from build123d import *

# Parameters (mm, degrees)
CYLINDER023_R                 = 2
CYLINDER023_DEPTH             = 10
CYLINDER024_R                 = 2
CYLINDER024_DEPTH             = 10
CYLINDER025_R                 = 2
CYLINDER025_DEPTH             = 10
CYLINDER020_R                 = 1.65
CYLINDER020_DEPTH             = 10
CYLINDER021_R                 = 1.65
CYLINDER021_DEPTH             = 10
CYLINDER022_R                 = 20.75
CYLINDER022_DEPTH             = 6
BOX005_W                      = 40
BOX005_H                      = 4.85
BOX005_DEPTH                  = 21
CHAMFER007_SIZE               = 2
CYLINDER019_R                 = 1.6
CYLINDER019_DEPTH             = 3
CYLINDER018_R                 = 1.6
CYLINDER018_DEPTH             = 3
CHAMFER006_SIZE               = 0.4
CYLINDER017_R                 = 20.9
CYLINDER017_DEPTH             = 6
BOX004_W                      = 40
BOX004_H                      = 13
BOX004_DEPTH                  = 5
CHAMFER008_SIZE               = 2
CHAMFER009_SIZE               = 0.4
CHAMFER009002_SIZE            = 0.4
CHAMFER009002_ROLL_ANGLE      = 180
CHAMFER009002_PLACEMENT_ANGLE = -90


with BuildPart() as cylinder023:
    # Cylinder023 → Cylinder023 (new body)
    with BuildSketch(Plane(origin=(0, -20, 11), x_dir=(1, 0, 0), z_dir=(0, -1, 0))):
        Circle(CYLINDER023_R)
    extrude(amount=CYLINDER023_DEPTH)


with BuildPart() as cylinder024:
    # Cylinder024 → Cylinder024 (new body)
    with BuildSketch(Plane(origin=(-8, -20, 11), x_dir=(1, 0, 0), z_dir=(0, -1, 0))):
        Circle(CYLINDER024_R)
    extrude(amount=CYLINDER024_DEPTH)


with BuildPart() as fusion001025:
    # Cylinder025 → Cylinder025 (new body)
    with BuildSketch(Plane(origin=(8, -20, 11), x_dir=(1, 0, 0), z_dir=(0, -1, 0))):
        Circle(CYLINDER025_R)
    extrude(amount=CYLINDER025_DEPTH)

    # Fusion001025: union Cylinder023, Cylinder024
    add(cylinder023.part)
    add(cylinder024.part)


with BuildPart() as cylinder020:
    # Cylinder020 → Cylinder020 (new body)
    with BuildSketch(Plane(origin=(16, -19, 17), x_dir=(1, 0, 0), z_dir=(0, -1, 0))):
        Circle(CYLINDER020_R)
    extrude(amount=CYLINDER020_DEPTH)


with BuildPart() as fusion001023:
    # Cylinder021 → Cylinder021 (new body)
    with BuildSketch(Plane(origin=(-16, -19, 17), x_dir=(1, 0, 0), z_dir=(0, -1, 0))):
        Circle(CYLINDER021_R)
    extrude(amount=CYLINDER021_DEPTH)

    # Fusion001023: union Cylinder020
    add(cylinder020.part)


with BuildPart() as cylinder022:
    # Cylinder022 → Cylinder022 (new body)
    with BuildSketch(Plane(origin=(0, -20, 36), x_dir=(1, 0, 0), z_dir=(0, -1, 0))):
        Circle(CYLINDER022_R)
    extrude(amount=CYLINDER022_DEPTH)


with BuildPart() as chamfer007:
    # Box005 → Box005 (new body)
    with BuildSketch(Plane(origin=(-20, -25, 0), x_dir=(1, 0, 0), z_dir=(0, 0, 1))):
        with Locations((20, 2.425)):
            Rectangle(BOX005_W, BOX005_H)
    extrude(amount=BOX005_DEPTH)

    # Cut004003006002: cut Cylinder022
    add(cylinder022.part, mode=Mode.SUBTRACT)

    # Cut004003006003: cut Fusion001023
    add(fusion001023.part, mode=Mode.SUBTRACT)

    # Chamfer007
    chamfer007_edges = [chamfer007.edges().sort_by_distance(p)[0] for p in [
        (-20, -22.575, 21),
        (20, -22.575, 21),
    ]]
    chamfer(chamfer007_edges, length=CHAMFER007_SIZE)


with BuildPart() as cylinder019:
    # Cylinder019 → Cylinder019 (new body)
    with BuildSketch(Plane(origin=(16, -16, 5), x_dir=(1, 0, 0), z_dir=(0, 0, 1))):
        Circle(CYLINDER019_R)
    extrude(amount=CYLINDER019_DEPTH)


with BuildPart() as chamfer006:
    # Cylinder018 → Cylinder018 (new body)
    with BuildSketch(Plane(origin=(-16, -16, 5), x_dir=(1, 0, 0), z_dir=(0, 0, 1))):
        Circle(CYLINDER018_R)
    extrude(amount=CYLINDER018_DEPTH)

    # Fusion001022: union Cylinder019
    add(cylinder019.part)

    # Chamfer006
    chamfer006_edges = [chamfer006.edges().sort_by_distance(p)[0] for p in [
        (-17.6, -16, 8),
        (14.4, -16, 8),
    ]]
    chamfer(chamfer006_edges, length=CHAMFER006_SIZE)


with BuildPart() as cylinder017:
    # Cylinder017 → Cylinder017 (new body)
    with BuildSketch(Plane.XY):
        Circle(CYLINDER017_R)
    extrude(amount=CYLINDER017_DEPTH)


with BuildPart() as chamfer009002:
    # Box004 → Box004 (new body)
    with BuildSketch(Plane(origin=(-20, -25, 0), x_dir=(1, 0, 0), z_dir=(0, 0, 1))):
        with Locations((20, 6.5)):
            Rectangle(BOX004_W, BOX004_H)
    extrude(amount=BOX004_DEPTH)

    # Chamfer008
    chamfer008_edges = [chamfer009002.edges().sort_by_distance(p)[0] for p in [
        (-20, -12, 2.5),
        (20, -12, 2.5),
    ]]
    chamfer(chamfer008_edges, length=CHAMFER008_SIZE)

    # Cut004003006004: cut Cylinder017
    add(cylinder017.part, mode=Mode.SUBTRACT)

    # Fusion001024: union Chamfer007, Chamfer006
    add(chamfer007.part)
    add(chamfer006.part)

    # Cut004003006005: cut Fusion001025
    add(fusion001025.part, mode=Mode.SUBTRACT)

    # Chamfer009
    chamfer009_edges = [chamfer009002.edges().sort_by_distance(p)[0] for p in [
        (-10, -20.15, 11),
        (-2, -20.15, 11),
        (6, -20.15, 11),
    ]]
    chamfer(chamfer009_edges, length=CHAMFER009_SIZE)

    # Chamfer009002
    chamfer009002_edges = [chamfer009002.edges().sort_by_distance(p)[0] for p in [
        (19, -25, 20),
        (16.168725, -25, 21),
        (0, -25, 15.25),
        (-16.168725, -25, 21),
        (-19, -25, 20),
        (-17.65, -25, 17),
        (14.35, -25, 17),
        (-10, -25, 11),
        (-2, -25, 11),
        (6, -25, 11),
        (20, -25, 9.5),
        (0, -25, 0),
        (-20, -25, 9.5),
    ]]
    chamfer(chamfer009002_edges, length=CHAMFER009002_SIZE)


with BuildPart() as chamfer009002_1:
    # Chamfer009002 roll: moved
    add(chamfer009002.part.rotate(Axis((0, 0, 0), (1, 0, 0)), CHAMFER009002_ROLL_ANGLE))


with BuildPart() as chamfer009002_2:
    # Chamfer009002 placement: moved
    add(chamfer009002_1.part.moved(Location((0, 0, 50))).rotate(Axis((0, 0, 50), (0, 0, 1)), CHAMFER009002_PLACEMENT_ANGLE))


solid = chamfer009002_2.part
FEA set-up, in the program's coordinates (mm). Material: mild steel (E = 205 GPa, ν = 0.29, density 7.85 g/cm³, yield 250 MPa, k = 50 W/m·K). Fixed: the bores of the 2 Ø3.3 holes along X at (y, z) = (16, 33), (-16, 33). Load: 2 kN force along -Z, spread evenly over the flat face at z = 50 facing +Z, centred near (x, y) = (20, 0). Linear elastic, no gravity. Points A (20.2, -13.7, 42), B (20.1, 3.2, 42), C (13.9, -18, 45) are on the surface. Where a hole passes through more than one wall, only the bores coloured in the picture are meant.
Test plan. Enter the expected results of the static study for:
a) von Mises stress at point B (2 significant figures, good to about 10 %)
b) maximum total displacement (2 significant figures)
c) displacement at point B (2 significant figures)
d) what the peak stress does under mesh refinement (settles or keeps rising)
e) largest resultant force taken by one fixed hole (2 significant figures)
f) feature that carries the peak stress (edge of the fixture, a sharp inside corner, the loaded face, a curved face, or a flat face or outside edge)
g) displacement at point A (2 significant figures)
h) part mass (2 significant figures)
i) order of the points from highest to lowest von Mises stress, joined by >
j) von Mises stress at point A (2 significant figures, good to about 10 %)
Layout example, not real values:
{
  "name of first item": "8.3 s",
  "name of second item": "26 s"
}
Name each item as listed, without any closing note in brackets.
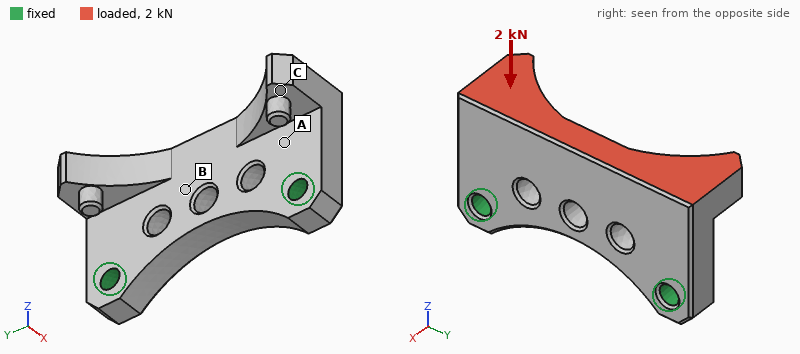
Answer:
{
  "von Mises stress at point B": "21 MPa",
  "maximum total displacement": "22 µm",
  "displacement at point B": "6.4 µm",
  "what the peak stress does under mesh refinement": "keeps rising",
  "largest resultant force taken by one fixed hole": "1.0 kN",
  "feature that carries the peak stress": "edge of the fixture",
  "displacement at point A": "5.3 µm",
  "part mass": "30 g",
  "order of the points from highest to lowest von Mises stress, joined by >": "A > B > C",
  "von Mises stress at point A": "55 MPa"
}
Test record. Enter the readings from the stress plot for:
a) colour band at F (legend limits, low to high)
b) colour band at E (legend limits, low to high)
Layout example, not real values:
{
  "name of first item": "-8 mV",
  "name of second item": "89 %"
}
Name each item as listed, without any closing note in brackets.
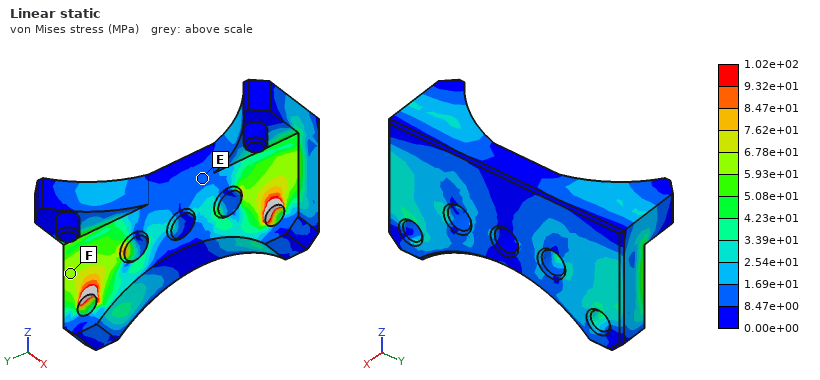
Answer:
{
  "colour band at F": "5.93e+01 to 6.78e+01 MPa",
  "colour band at E": "8.47e+00 to 1.69e+01 MPa"
}
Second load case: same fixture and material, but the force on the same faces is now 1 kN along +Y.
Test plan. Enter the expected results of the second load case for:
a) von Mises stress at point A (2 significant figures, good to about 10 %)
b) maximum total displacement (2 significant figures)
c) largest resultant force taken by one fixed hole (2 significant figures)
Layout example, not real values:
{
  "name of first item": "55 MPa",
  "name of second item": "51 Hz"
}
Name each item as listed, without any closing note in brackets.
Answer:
{
  "von Mises stress at point A": "15 MPa",
  "maximum total displacement": "5.3 µm",
  "largest resultant force taken by one fixed hole": "690 N"
}
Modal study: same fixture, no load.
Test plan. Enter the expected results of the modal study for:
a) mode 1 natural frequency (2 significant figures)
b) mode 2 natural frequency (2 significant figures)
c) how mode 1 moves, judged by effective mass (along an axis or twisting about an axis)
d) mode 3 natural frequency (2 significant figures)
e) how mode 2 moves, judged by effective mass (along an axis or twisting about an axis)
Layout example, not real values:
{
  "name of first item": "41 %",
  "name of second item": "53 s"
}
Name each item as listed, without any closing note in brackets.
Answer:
{
  "mode 1 natural frequency": "7500 Hz",
  "mode 2 natural frequency": "12 kHz",
  "how mode 1 moves, judged by effective mass": "along X",
  "mode 3 natural frequency": "17 kHz",
  "how mode 2 moves, judged by effective mass": "twisting about Z"
}
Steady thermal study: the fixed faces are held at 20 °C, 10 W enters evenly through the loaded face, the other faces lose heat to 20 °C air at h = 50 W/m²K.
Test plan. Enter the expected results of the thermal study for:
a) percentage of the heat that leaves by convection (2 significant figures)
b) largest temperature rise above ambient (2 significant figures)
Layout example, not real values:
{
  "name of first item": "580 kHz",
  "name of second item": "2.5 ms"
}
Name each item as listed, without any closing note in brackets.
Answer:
{
  "percentage of the heat that leaves by convection": "14 %",
  "largest temperature rise above ambient": "24 K"
}
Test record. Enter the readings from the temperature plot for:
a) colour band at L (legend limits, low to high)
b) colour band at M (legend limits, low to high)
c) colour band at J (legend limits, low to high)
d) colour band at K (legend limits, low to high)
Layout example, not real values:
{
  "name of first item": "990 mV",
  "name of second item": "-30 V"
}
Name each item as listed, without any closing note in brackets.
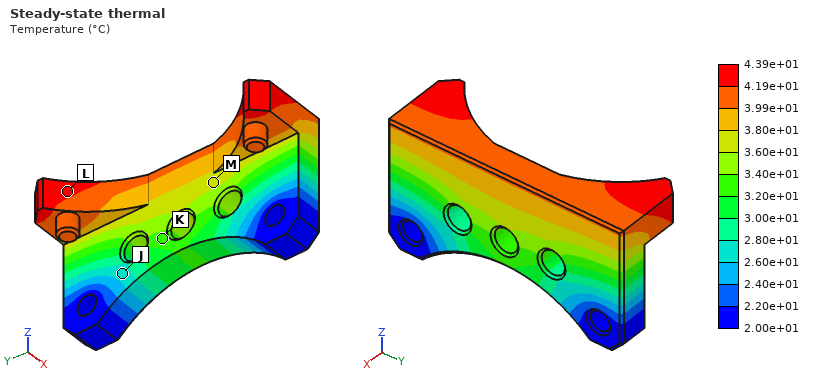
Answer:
{
  "colour band at L": "4.19e+01 to 4.39e+01 °C",
  "colour band at M": "3.60e+01 to 3.80e+01 °C",
  "colour band at J": "2.60e+01 to 2.80e+01 °C",
  "colour band at K": "3.20e+01 to 3.40e+01 °C"
}
